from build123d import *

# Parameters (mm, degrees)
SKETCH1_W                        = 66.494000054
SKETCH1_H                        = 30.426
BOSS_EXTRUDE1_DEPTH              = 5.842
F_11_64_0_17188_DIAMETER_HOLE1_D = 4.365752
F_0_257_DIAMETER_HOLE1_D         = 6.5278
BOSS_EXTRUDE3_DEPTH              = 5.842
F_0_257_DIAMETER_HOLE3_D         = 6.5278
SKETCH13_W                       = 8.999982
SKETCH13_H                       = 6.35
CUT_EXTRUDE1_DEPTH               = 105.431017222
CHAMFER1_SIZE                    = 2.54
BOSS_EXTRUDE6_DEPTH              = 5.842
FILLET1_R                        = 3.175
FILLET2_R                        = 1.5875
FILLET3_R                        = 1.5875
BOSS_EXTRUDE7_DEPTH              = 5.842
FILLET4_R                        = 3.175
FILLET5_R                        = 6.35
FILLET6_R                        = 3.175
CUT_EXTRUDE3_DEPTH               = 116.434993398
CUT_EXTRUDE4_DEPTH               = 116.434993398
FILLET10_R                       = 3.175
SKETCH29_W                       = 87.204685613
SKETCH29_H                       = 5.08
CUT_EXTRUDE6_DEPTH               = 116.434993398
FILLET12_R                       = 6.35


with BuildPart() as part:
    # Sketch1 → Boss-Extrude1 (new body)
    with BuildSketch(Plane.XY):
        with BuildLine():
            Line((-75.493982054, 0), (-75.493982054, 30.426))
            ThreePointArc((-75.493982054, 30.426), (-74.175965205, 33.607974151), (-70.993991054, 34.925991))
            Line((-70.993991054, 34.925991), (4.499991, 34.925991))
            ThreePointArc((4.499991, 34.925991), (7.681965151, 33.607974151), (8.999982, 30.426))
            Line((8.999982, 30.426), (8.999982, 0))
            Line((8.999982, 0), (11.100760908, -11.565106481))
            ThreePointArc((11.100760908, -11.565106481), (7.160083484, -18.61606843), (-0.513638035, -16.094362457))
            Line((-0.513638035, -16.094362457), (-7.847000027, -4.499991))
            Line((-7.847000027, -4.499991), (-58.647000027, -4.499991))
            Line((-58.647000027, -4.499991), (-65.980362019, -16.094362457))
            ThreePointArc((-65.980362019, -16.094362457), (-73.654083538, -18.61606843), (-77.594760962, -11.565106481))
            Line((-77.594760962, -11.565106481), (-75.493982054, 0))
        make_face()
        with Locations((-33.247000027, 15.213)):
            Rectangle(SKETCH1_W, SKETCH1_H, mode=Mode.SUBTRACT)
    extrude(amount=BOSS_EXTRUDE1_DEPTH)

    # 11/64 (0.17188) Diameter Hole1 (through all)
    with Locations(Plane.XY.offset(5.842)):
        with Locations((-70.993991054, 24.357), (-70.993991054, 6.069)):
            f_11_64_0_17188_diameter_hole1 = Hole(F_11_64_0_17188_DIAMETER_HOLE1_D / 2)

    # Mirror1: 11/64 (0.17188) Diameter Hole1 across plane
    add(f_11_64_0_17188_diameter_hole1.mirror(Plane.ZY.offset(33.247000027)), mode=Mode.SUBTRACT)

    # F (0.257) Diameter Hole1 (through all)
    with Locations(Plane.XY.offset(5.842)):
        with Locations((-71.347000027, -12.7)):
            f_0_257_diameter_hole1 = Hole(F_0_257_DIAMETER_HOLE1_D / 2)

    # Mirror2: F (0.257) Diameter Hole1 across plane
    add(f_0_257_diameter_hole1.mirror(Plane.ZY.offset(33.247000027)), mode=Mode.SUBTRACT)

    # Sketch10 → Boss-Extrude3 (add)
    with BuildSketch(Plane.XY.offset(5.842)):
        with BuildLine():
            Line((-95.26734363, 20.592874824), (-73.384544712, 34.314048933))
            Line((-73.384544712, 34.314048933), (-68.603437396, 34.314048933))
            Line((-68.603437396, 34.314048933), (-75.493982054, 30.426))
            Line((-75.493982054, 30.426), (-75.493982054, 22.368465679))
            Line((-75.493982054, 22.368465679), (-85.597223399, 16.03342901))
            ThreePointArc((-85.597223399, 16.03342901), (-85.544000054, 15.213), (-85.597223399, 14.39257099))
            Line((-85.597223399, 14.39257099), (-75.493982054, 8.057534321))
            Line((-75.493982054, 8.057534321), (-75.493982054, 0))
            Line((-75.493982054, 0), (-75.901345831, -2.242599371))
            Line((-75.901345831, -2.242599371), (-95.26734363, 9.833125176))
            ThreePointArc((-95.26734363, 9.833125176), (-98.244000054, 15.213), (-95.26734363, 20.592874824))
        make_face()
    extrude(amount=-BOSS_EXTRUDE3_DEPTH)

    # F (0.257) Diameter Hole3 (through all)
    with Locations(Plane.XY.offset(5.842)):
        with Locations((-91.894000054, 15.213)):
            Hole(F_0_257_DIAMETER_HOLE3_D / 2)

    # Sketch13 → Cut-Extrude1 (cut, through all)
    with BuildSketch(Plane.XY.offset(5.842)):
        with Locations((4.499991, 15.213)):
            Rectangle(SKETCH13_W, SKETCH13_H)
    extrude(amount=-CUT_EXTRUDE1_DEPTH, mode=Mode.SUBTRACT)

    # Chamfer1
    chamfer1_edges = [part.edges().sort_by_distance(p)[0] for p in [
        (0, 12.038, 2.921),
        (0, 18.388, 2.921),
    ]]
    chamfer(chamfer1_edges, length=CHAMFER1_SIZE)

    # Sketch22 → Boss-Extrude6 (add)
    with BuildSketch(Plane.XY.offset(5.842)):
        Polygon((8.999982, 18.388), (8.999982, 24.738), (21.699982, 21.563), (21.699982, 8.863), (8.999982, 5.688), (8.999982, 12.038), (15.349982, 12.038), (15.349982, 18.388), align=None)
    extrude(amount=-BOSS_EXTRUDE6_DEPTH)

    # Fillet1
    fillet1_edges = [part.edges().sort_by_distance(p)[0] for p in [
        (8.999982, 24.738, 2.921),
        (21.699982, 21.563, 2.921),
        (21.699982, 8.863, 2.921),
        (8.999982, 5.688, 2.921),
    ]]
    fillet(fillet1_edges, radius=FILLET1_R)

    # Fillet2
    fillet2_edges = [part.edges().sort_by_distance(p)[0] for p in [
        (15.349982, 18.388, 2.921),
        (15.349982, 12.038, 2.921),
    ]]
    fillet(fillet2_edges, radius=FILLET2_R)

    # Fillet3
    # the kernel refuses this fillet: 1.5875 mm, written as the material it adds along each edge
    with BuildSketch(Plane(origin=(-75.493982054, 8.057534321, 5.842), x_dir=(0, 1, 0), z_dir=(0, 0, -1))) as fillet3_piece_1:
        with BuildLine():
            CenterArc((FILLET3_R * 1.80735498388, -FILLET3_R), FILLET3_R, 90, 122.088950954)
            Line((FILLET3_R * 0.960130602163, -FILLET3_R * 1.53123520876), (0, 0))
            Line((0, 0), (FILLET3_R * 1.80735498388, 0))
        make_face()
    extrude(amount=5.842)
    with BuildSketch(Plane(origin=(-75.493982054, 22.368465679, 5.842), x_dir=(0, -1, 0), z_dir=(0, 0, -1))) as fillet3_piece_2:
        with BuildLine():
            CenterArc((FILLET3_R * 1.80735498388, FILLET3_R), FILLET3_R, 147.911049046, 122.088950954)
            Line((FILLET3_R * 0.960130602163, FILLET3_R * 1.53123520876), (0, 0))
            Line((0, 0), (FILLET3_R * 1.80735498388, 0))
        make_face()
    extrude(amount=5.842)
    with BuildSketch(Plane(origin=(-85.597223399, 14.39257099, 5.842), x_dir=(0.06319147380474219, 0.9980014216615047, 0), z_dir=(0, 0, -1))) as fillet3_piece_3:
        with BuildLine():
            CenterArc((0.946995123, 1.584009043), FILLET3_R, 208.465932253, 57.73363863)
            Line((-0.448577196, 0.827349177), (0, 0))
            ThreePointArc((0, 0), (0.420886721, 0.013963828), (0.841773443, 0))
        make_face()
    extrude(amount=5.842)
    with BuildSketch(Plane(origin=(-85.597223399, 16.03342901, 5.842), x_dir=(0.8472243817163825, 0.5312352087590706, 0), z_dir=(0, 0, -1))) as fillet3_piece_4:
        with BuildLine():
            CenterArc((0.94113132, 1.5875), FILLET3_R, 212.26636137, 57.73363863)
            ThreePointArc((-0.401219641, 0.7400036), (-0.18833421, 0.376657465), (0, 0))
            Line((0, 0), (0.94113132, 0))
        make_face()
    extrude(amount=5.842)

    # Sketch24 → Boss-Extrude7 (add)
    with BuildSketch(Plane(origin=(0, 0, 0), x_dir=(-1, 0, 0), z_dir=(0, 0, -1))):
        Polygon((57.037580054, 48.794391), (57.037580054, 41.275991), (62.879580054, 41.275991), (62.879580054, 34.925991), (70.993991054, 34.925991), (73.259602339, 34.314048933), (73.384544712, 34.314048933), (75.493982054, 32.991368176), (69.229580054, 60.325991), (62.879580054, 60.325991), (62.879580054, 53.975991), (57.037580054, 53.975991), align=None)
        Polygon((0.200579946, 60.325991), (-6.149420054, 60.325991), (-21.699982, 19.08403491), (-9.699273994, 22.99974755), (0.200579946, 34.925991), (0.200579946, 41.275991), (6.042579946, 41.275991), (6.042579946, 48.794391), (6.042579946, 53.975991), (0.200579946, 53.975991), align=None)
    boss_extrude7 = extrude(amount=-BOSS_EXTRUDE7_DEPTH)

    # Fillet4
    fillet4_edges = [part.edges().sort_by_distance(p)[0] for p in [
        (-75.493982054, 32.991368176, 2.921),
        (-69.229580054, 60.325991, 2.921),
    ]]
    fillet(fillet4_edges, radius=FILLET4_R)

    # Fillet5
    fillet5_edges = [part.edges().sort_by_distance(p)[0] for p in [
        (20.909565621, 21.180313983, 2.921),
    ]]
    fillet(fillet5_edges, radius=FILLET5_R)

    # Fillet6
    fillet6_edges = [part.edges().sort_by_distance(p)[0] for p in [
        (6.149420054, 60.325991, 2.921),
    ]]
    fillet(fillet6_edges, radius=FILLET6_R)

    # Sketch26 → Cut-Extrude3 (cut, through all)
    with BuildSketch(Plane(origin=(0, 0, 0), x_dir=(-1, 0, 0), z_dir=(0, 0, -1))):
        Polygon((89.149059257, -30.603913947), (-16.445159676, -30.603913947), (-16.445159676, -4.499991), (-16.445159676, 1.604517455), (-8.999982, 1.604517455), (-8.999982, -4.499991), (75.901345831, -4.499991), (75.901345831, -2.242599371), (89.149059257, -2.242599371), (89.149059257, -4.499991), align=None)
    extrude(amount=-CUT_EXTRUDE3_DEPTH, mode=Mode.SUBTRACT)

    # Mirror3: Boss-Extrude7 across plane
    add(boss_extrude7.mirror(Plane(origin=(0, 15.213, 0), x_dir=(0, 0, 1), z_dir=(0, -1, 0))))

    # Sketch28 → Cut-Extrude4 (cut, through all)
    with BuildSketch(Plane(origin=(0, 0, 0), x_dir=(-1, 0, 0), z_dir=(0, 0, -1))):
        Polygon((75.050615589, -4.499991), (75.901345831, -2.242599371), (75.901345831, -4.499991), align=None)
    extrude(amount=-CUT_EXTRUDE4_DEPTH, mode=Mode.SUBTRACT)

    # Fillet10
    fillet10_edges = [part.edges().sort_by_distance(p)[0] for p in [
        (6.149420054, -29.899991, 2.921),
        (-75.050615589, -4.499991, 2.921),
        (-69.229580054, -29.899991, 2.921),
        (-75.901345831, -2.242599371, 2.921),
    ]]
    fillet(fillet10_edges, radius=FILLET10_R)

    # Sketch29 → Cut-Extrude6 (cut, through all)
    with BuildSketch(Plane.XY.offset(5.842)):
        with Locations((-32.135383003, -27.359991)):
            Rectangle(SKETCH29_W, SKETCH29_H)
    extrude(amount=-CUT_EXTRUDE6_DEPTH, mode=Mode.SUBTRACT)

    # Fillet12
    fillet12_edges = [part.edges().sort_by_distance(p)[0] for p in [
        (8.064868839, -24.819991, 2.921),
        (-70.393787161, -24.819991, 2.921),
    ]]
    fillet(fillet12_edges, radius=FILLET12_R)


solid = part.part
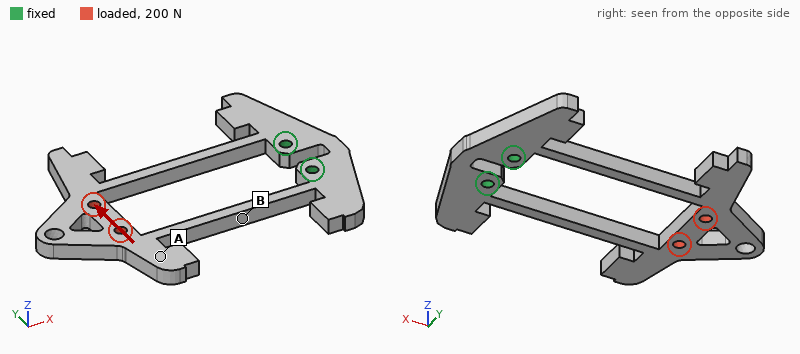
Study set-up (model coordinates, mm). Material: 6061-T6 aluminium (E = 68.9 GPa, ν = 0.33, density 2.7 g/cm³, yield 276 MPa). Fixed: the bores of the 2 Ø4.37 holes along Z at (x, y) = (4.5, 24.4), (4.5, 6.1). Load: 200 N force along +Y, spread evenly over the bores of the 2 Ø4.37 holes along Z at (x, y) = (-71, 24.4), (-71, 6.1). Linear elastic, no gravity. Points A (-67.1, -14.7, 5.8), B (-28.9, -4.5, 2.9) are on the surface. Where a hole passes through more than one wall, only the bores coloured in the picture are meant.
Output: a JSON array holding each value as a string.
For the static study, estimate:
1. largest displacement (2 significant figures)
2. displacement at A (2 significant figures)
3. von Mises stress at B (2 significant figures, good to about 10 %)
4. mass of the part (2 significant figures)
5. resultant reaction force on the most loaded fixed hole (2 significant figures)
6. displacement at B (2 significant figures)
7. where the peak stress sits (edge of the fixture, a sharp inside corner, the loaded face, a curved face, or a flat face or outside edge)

["0.94 mm", "0.91 mm", "27 MPa", "50 g", "420 N", "0.39 mm", "a flat face or outside edge"]
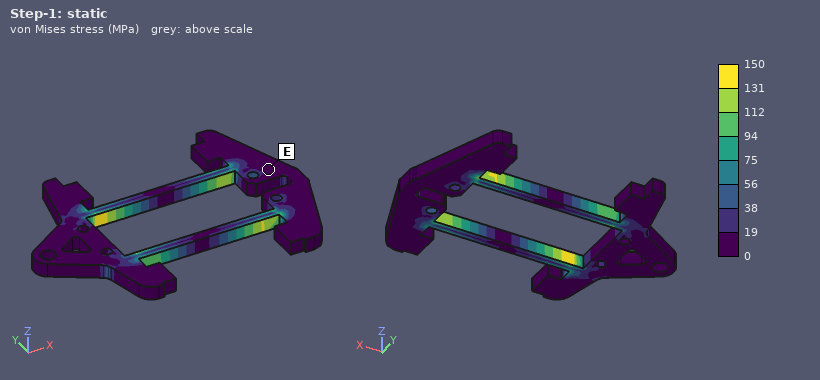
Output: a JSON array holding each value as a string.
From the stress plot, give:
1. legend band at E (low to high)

["0 to 19 MPa"]
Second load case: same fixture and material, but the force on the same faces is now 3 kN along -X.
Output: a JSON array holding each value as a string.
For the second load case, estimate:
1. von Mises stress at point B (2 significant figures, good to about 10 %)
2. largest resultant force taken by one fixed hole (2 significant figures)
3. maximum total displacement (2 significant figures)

["53 MPa", "1.6 kN", "88 µm"]
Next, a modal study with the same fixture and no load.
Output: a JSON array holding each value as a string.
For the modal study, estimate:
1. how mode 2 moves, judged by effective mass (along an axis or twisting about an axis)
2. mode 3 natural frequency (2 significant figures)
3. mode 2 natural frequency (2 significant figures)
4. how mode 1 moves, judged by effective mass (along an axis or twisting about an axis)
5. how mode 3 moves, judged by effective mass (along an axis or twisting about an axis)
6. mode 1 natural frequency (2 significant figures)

["along Y", "600 Hz", "480 Hz", "along Z", "twisting about X", "270 Hz"]
